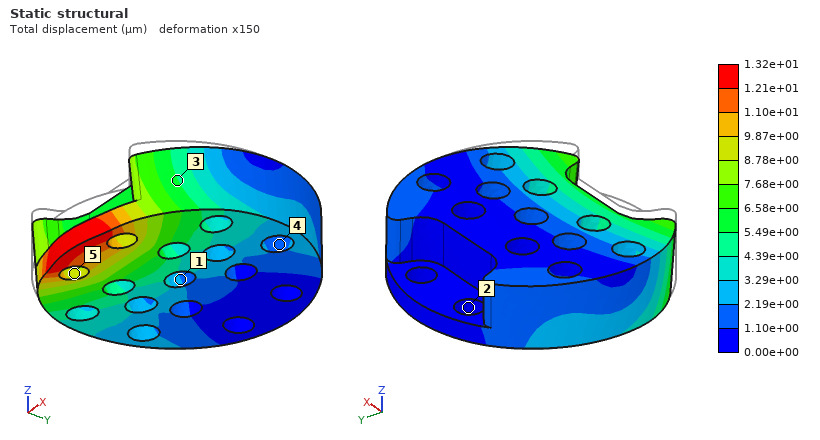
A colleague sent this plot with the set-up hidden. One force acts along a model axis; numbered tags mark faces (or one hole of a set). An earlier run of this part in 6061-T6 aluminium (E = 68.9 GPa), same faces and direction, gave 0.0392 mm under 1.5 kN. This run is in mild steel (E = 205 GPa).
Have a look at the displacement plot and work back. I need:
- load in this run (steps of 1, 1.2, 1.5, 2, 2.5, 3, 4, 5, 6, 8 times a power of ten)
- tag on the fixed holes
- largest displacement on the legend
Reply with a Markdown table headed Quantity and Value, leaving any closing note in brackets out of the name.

| Quantity | Value |
|---|---|
| load in this run | 1.5 kN |
| tag on the fixed holes | 2 |
| largest displacement on the legend | 1.32e+01 µm |
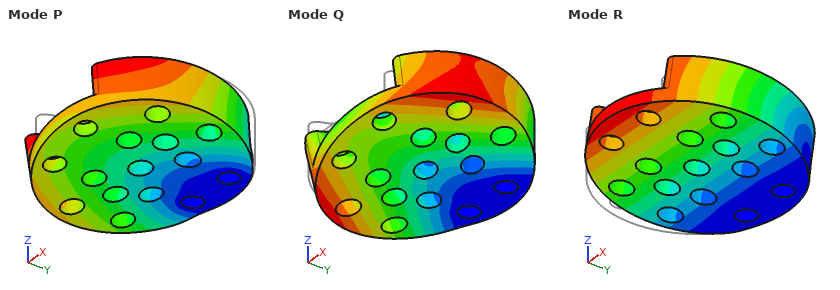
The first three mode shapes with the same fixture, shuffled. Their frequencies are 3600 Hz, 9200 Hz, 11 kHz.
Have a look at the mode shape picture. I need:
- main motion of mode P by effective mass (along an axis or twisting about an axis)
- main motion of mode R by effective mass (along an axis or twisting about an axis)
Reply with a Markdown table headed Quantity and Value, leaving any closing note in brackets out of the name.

| Quantity | Value |
|---|---|
| main motion of mode P by effective mass | along X |
| main motion of mode R by effective mass | along Z |
